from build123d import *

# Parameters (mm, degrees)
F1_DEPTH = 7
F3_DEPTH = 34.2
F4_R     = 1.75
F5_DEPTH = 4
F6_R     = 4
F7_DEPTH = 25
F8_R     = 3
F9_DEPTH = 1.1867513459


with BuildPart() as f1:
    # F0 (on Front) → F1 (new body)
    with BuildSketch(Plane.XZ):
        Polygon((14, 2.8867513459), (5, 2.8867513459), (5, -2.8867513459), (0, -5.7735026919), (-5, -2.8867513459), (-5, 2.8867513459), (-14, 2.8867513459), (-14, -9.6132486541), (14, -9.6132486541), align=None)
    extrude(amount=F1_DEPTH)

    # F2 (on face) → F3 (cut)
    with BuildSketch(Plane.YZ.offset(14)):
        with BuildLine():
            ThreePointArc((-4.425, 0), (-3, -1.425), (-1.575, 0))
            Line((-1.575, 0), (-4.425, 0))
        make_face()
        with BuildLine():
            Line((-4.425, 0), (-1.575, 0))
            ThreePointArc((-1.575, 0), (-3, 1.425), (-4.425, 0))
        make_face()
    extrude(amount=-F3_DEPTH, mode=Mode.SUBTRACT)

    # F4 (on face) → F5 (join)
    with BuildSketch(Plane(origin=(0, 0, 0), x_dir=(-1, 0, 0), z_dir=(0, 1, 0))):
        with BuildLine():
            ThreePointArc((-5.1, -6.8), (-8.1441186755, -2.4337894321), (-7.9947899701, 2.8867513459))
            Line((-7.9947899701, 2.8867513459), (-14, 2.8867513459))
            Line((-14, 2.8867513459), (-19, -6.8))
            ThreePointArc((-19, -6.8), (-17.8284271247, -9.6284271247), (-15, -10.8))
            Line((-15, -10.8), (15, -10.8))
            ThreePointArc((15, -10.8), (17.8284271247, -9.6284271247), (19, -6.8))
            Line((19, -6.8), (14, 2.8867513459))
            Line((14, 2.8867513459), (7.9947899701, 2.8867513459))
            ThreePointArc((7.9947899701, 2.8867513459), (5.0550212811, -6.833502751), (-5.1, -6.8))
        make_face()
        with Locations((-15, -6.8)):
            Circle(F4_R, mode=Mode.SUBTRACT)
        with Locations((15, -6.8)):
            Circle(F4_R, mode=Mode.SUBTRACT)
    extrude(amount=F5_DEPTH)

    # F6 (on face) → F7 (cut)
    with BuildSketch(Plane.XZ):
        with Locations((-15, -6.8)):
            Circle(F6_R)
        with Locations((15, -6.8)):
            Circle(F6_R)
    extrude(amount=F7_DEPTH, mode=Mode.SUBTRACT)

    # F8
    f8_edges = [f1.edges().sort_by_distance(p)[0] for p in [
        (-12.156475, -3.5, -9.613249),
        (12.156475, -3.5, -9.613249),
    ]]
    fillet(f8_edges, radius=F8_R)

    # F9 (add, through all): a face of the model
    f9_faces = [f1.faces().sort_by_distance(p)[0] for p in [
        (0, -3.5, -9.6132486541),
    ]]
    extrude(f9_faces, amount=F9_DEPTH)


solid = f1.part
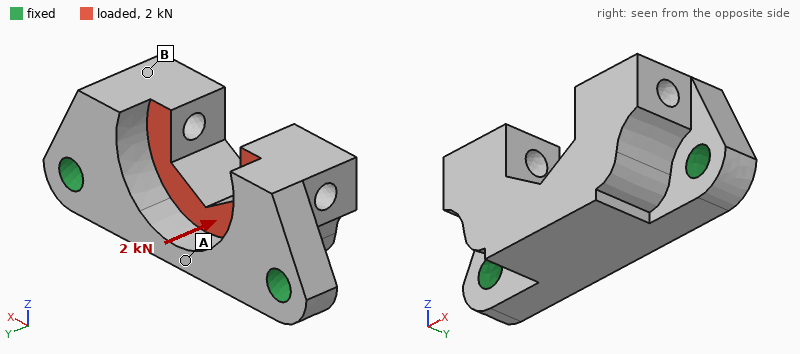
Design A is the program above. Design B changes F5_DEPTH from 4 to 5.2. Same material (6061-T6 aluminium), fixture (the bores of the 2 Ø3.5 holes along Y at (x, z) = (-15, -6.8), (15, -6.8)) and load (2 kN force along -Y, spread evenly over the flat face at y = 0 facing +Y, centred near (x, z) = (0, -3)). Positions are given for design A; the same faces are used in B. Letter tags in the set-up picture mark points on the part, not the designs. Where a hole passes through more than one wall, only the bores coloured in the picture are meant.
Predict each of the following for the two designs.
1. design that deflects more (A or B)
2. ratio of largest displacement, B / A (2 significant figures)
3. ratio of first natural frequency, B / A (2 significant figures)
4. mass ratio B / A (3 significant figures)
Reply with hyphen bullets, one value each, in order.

- A
- 0.68
- 1.2
- 1.12
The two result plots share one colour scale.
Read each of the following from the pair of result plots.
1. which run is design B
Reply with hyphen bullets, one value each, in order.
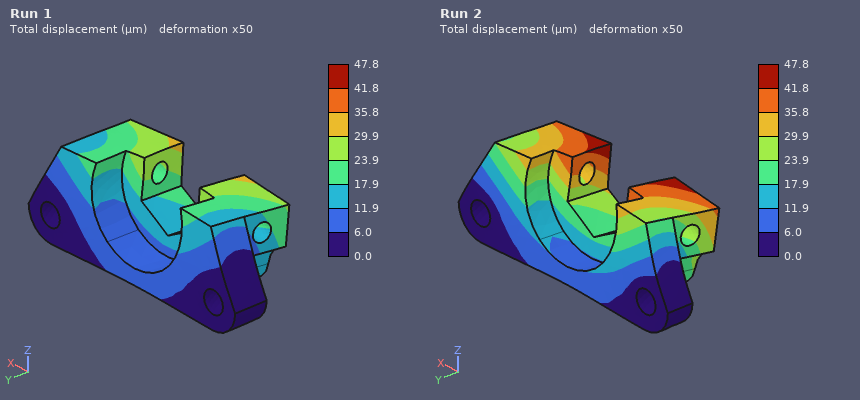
- Run 1
